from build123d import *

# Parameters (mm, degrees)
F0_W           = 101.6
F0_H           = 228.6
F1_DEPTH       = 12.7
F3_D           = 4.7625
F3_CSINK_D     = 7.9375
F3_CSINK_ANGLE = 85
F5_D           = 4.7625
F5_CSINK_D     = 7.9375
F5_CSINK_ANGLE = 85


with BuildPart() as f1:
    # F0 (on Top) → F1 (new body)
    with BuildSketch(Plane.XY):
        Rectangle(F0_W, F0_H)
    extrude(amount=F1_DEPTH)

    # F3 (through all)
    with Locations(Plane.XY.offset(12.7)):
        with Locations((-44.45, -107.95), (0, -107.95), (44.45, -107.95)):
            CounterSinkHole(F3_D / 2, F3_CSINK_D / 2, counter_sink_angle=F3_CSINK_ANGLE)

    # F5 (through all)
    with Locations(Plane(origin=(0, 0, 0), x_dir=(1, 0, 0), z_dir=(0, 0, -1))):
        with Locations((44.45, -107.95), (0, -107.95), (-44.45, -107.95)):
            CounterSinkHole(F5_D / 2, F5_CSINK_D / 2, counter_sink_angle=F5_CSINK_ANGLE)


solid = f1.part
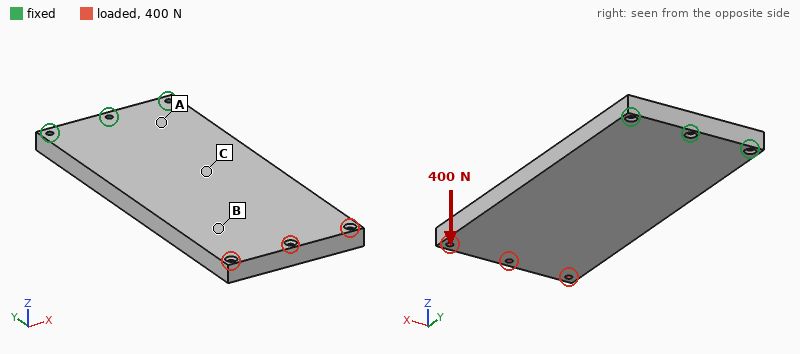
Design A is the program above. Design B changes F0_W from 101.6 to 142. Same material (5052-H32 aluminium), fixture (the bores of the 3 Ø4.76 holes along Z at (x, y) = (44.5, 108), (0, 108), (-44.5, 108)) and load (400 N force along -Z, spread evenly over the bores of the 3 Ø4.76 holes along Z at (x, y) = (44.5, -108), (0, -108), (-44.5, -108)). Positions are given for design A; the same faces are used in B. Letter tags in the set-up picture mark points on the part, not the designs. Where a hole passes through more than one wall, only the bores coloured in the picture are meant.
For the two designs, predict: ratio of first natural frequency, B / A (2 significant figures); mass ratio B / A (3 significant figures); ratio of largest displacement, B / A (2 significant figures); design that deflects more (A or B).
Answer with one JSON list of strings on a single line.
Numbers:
["0.98", "1.40", "0.74", "A"]
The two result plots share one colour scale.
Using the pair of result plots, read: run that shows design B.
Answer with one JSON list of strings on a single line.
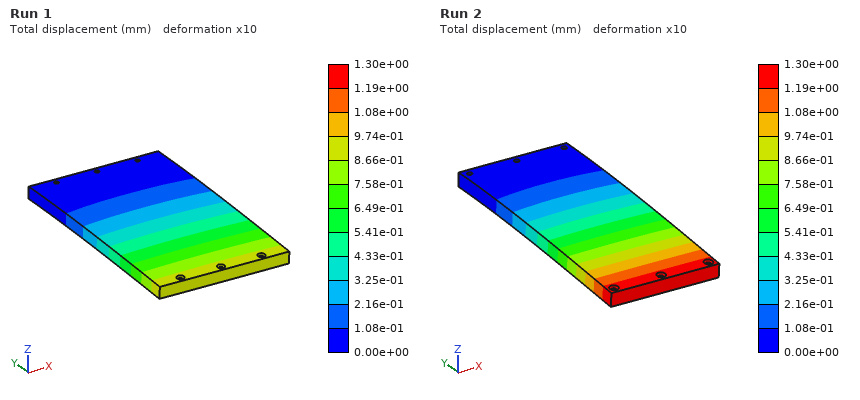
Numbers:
["Run 1"]
